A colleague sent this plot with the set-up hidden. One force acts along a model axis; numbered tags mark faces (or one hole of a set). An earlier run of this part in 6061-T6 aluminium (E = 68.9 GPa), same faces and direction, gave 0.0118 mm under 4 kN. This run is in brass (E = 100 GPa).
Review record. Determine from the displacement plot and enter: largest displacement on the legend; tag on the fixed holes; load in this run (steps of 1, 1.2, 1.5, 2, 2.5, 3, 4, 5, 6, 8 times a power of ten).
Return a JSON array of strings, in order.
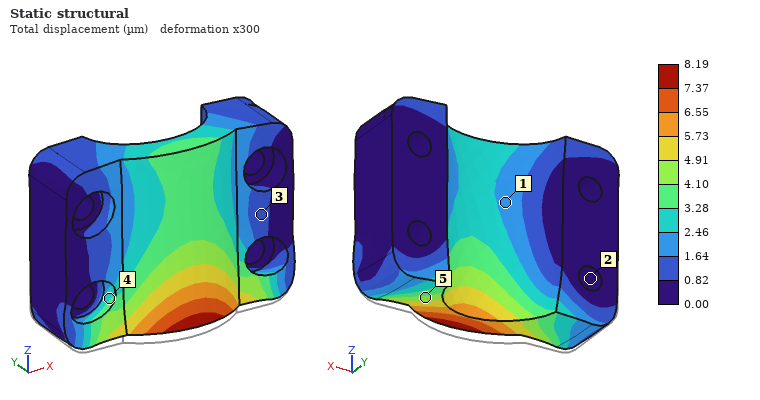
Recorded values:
["8.19 µm", "2", "4 kN"]
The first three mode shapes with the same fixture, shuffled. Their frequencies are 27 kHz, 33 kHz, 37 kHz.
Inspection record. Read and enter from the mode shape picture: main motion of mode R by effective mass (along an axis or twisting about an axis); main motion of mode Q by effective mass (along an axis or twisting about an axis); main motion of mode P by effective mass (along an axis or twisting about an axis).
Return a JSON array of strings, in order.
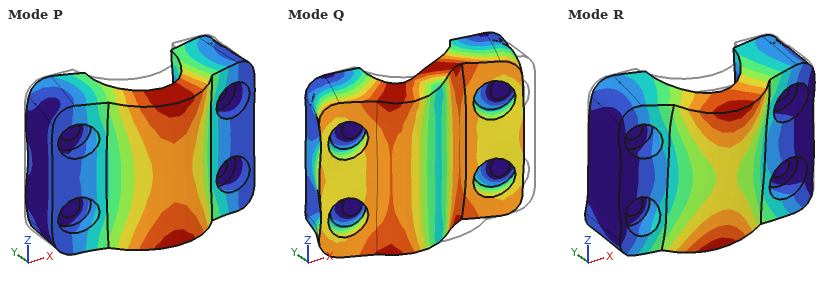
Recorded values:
["along Z", "along X", "along Y"]
